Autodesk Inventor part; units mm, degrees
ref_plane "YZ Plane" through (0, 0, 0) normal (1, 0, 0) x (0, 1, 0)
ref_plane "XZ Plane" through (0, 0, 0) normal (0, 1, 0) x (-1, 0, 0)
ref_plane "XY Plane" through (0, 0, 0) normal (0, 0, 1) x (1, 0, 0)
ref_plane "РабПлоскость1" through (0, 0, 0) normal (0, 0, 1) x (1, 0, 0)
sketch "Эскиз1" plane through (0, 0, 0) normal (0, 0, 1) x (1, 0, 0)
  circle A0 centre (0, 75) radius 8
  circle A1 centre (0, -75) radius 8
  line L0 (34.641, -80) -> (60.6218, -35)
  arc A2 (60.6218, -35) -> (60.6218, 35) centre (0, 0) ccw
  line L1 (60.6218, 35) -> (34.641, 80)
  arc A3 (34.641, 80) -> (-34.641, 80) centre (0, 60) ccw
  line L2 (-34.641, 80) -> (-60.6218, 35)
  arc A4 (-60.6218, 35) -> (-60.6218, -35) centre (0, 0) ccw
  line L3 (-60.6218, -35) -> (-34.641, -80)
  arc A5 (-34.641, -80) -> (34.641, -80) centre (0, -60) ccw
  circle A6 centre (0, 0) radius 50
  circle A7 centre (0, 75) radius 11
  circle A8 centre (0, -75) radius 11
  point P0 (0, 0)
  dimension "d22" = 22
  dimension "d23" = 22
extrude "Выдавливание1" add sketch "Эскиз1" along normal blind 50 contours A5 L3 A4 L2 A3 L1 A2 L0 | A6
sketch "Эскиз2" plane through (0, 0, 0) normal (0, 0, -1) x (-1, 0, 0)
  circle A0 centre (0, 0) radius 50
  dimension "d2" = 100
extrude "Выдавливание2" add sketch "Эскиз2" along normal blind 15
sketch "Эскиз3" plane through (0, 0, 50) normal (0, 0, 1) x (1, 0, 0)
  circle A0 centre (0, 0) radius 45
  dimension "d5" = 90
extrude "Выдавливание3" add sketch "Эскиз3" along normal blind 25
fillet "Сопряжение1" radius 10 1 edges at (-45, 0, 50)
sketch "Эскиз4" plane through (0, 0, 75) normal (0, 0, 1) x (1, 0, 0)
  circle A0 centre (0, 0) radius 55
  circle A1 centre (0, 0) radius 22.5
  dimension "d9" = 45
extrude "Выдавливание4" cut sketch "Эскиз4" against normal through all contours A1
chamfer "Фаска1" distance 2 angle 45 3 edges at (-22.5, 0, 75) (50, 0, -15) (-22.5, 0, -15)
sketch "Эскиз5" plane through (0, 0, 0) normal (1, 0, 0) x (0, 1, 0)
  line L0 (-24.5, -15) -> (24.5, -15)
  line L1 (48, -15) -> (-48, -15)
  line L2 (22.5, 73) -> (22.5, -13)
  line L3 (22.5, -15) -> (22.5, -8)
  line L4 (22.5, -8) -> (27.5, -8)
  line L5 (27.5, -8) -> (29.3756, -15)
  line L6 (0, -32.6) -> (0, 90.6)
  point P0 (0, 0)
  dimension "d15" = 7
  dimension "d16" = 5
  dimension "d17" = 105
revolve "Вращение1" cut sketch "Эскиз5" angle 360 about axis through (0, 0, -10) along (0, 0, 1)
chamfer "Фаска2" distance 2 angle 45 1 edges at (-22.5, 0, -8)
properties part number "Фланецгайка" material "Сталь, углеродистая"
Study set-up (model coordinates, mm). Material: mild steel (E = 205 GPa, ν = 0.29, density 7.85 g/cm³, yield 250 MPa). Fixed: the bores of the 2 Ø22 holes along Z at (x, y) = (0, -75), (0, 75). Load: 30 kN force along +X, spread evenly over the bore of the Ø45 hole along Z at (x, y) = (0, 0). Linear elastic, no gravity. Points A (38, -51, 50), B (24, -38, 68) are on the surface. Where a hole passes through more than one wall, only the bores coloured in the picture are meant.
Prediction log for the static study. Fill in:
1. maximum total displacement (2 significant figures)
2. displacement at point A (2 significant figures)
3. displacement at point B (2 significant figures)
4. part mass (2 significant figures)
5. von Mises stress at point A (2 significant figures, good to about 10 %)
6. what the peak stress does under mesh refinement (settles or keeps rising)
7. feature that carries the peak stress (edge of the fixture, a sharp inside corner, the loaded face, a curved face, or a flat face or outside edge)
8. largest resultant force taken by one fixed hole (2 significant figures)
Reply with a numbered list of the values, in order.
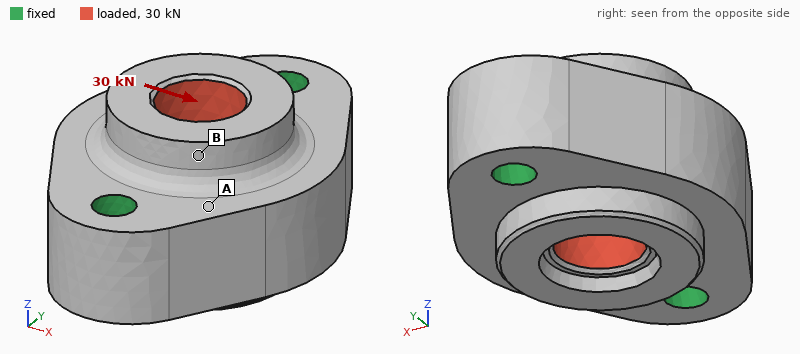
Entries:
1. 4.6 µm
2. 2.1 µm
3. 3.6 µm
4. 8.6 kg
5. 5.4 MPa
6. keeps rising
7. edge of the fixture
8. 15 kN
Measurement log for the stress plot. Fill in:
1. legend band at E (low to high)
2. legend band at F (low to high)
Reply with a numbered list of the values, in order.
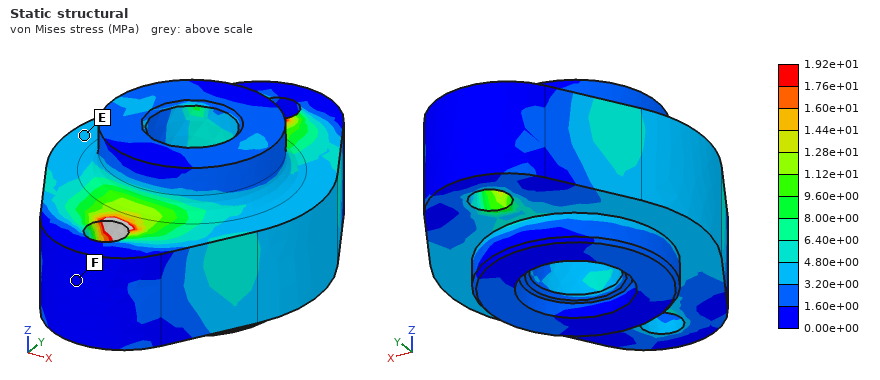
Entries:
1. 3.20e+00 to 4.80e+00 MPa
2. 0.00e+00 to 1.60e+00 MPa
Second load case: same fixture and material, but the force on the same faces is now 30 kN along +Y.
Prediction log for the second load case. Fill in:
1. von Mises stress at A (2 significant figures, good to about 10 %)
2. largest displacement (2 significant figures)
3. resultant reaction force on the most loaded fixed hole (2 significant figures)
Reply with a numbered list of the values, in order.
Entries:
1. 1.9 MPa
2. 1.9 µm
3. 15 kN
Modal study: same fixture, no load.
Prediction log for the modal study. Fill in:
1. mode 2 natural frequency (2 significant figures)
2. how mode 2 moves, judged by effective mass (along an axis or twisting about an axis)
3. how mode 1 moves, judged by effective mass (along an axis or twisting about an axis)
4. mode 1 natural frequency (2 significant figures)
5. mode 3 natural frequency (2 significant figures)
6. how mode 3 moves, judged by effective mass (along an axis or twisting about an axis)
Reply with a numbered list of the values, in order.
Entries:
1. 5800 Hz
2. along Z
3. twisting about Y
4. 4600 Hz
5. 7600 Hz
6. along X
